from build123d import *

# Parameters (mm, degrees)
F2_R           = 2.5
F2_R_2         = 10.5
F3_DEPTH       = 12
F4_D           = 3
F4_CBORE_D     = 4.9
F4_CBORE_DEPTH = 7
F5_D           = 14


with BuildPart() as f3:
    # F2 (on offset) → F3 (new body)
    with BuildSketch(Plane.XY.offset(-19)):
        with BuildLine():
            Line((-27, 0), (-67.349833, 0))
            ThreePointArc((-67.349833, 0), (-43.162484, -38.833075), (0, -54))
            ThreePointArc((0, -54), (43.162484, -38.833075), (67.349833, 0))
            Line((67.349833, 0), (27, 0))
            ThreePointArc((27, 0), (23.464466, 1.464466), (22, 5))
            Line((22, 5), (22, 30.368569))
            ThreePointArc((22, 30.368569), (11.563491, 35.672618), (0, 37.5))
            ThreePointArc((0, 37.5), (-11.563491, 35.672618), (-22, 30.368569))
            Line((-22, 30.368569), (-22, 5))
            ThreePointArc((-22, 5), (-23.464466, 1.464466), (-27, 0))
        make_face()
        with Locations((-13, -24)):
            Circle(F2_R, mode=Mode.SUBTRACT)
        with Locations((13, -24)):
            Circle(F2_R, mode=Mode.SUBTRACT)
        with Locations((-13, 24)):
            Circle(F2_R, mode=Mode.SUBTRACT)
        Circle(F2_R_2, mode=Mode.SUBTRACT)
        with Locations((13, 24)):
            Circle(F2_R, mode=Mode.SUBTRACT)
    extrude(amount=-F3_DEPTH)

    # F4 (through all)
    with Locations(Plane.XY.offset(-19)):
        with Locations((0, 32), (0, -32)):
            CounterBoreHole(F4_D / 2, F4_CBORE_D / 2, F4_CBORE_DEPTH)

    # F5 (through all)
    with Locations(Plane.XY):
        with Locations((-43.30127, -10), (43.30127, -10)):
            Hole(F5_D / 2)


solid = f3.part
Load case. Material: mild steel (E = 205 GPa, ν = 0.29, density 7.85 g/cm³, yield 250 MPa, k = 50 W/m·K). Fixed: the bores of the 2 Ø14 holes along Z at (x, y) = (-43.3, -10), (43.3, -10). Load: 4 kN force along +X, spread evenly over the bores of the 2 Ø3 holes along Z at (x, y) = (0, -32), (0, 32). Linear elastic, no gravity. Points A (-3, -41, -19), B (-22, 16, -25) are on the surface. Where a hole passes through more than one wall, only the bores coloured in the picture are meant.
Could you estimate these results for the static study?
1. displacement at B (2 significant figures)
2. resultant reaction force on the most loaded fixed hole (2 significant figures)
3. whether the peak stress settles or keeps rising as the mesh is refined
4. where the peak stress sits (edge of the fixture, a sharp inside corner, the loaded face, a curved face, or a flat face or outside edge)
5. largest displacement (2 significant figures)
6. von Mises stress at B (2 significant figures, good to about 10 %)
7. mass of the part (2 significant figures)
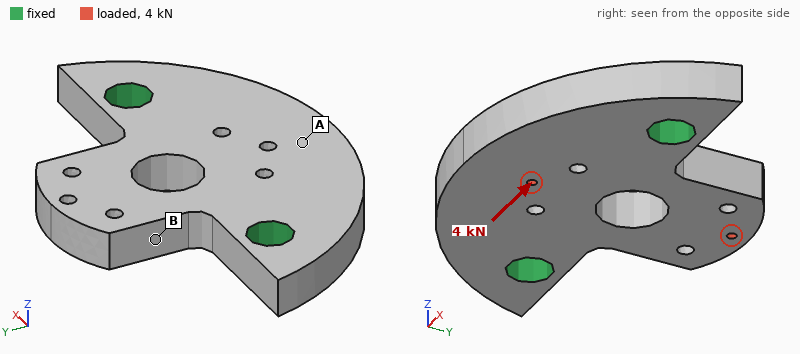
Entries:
4.5 µm
2.1 kN
keeps rising
a sharp inside corner
8.1 µm
7.9 MPa
590 g
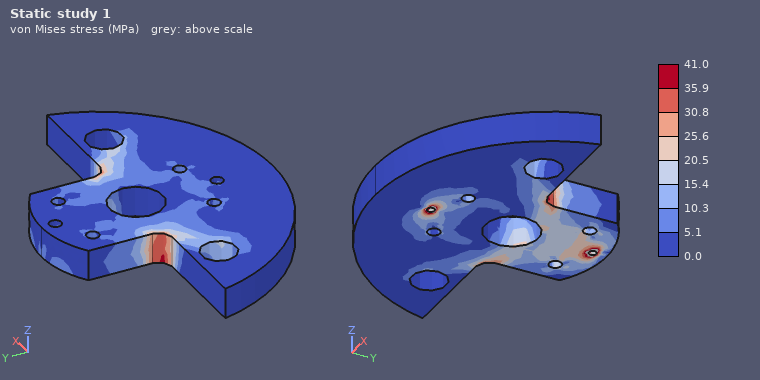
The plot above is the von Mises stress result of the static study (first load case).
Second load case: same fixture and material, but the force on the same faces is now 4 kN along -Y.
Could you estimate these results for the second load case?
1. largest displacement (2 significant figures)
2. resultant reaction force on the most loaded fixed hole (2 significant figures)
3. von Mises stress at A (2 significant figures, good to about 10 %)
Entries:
15 µm
2.1 kN
7.6 MPa
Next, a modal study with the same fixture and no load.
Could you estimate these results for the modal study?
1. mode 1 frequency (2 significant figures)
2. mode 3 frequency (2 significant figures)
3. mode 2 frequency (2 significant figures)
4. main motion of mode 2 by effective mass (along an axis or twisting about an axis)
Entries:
3000 Hz
9200 Hz
5000 Hz
along Z
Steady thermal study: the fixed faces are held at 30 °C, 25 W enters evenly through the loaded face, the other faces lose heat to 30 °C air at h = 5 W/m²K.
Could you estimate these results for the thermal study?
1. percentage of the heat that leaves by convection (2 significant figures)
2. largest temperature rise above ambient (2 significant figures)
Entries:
4.9 %
50 K
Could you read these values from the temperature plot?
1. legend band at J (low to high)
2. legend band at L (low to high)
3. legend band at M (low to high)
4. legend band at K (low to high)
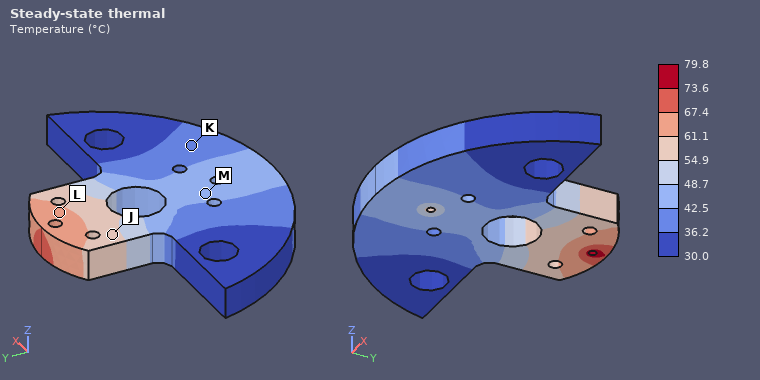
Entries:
54.9 to 61.1 °C
61.1 to 67.4 °C
42.5 to 48.7 °C
36.2 to 42.5 °C
